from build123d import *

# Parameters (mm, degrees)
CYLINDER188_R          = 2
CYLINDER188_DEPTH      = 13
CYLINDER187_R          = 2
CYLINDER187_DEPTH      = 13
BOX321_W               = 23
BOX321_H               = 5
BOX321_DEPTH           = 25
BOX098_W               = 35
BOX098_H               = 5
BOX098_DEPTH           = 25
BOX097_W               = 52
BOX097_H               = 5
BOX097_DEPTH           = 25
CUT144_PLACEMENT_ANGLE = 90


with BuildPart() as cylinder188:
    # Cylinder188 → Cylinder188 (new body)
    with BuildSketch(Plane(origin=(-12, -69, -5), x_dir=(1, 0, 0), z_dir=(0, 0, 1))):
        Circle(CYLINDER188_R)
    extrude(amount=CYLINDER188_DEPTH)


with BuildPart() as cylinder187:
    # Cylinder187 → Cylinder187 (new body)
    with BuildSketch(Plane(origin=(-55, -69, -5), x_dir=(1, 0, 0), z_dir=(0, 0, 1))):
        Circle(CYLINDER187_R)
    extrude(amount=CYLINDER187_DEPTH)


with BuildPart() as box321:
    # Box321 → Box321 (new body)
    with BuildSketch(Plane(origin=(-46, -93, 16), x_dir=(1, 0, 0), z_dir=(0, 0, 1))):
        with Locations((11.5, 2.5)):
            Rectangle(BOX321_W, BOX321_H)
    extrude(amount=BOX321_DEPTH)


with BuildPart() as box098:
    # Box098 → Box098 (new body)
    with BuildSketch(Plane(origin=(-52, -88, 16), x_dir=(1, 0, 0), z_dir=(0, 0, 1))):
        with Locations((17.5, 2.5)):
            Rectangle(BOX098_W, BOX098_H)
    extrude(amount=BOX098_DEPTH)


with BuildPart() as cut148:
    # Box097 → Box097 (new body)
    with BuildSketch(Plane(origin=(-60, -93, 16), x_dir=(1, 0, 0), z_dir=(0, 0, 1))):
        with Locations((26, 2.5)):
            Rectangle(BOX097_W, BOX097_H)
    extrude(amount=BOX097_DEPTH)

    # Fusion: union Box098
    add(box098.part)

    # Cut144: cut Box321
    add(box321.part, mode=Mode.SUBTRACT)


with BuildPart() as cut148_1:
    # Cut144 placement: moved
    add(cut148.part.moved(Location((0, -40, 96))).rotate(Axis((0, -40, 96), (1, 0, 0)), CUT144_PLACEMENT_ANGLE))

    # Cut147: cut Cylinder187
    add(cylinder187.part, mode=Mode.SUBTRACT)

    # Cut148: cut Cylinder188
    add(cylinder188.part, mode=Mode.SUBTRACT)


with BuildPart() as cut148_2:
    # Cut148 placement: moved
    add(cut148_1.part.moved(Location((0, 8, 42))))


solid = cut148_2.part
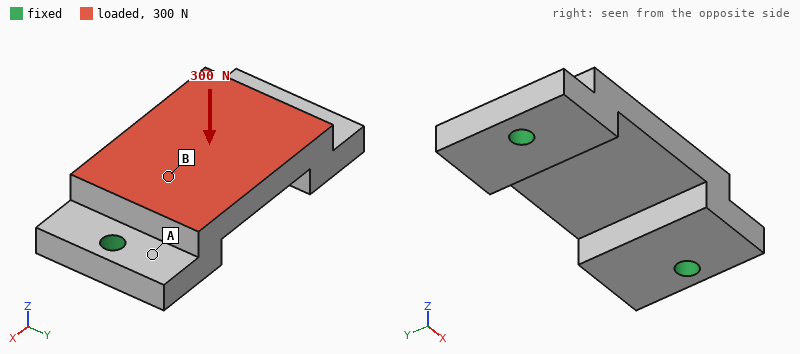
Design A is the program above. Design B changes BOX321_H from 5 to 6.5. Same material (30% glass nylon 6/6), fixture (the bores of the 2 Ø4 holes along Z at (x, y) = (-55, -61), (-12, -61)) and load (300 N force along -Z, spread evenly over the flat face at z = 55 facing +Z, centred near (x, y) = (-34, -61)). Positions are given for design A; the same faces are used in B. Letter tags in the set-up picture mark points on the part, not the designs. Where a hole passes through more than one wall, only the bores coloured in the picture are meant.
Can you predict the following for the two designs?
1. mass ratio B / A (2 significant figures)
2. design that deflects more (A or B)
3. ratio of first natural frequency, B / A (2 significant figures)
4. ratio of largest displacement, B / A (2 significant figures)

0.95
B
1.0
1.1
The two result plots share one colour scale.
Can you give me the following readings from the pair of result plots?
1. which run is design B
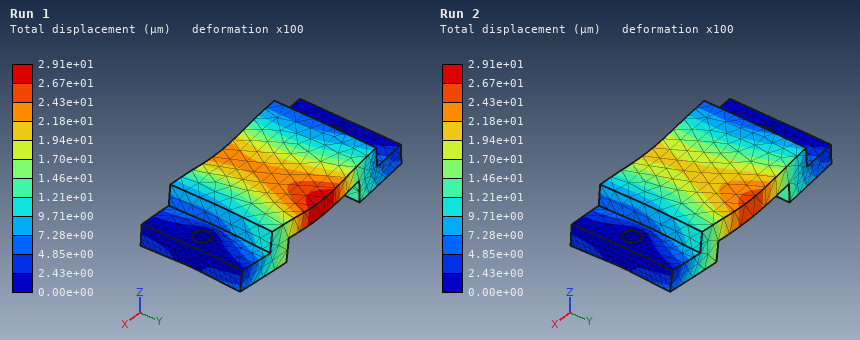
Run 1
